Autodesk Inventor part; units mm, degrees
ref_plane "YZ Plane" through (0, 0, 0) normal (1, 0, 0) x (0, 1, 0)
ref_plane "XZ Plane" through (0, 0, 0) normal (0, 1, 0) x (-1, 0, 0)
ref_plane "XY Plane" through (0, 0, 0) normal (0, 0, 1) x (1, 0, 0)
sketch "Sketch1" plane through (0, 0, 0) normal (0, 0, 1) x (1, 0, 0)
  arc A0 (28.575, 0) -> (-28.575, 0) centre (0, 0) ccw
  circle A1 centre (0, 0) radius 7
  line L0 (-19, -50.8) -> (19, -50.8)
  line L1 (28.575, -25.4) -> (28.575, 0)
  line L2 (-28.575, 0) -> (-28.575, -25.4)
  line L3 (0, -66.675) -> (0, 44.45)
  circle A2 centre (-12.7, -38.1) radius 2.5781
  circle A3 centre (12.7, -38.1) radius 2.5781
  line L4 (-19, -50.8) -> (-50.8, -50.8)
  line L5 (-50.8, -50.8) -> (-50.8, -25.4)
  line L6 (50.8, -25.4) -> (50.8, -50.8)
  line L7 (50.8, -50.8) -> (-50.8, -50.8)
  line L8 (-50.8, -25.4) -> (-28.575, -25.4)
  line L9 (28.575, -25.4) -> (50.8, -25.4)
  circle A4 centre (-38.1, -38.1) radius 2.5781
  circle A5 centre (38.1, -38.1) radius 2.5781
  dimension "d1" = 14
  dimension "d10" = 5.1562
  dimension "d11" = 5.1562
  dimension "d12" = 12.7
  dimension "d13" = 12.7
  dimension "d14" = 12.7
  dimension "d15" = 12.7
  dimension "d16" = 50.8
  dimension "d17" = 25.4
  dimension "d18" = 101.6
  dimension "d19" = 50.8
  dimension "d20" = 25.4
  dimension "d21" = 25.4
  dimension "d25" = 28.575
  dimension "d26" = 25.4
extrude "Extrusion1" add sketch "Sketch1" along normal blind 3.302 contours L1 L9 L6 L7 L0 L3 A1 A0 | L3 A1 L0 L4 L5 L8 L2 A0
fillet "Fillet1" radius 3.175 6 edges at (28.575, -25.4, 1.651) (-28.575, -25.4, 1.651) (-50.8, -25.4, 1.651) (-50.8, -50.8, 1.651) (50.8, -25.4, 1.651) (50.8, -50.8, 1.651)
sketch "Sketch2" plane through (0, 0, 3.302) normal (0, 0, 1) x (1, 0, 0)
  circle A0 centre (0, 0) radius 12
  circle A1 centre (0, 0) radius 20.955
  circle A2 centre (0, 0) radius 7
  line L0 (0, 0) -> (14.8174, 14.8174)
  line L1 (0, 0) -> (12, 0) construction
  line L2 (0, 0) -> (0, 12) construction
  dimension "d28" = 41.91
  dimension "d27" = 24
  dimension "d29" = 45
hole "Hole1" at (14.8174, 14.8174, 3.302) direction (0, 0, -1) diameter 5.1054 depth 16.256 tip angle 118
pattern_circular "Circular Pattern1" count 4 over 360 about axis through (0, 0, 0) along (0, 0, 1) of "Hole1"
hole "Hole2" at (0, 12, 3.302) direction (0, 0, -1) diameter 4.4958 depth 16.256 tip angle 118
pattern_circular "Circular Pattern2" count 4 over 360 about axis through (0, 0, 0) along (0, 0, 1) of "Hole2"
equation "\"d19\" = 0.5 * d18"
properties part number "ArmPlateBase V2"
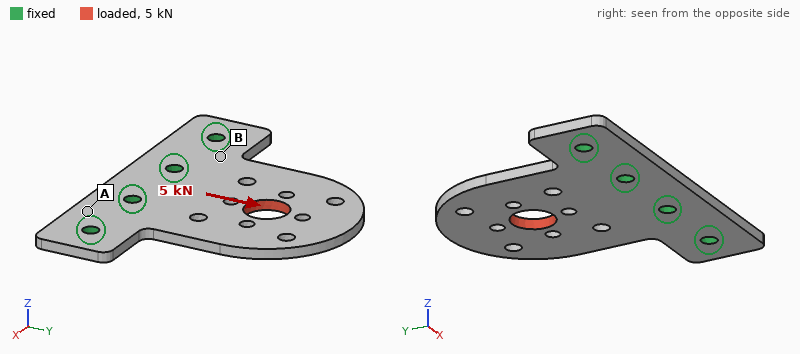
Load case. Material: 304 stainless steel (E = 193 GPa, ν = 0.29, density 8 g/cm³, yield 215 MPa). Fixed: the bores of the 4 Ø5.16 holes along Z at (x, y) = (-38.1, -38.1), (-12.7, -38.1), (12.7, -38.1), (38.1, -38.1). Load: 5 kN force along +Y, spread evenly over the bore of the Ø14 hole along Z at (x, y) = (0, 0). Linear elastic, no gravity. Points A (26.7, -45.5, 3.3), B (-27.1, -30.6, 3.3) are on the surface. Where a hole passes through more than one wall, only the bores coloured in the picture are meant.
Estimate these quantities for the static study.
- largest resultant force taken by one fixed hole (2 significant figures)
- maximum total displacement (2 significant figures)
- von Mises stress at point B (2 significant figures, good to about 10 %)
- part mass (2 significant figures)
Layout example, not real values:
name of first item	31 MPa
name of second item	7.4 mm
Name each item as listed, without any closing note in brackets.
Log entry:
largest resultant force taken by one fixed hole	2.0 kN
maximum total displacement	11 µm
von Mises stress at point B	17 MPa
part mass	130 g
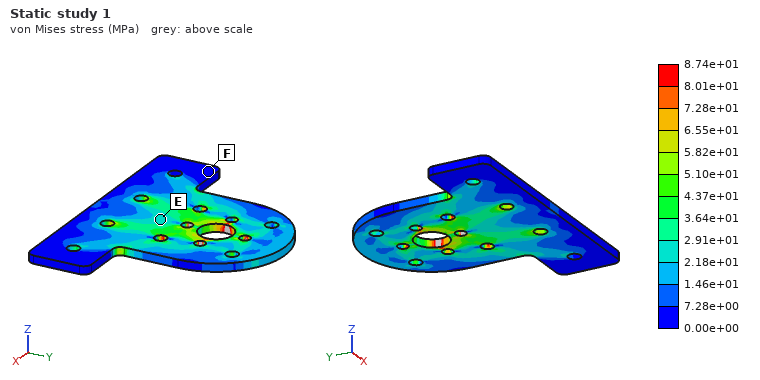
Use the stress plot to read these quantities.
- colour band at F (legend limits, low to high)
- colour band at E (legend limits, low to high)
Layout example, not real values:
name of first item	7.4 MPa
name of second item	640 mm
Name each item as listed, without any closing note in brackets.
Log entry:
colour band at F	0.00e+00 to 7.28e+00 MPa
colour band at E	2.18e+01 to 2.91e+01 MPa
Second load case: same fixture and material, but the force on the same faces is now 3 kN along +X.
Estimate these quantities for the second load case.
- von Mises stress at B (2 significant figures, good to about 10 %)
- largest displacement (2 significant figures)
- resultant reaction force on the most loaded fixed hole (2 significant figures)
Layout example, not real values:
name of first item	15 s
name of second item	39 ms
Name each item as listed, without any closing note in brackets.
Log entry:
von Mises stress at B	31 MPa
largest displacement	22 µm
resultant reaction force on the most loaded fixed hole	1.4 kN
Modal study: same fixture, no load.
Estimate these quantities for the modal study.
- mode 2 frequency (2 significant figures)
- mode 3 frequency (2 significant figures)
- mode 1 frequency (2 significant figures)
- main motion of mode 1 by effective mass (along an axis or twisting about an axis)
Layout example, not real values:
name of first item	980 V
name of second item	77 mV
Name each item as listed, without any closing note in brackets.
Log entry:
mode 2 frequency	2100 Hz
mode 3 frequency	3900 Hz
mode 1 frequency	760 Hz
main motion of mode 1 by effective mass	along Z
